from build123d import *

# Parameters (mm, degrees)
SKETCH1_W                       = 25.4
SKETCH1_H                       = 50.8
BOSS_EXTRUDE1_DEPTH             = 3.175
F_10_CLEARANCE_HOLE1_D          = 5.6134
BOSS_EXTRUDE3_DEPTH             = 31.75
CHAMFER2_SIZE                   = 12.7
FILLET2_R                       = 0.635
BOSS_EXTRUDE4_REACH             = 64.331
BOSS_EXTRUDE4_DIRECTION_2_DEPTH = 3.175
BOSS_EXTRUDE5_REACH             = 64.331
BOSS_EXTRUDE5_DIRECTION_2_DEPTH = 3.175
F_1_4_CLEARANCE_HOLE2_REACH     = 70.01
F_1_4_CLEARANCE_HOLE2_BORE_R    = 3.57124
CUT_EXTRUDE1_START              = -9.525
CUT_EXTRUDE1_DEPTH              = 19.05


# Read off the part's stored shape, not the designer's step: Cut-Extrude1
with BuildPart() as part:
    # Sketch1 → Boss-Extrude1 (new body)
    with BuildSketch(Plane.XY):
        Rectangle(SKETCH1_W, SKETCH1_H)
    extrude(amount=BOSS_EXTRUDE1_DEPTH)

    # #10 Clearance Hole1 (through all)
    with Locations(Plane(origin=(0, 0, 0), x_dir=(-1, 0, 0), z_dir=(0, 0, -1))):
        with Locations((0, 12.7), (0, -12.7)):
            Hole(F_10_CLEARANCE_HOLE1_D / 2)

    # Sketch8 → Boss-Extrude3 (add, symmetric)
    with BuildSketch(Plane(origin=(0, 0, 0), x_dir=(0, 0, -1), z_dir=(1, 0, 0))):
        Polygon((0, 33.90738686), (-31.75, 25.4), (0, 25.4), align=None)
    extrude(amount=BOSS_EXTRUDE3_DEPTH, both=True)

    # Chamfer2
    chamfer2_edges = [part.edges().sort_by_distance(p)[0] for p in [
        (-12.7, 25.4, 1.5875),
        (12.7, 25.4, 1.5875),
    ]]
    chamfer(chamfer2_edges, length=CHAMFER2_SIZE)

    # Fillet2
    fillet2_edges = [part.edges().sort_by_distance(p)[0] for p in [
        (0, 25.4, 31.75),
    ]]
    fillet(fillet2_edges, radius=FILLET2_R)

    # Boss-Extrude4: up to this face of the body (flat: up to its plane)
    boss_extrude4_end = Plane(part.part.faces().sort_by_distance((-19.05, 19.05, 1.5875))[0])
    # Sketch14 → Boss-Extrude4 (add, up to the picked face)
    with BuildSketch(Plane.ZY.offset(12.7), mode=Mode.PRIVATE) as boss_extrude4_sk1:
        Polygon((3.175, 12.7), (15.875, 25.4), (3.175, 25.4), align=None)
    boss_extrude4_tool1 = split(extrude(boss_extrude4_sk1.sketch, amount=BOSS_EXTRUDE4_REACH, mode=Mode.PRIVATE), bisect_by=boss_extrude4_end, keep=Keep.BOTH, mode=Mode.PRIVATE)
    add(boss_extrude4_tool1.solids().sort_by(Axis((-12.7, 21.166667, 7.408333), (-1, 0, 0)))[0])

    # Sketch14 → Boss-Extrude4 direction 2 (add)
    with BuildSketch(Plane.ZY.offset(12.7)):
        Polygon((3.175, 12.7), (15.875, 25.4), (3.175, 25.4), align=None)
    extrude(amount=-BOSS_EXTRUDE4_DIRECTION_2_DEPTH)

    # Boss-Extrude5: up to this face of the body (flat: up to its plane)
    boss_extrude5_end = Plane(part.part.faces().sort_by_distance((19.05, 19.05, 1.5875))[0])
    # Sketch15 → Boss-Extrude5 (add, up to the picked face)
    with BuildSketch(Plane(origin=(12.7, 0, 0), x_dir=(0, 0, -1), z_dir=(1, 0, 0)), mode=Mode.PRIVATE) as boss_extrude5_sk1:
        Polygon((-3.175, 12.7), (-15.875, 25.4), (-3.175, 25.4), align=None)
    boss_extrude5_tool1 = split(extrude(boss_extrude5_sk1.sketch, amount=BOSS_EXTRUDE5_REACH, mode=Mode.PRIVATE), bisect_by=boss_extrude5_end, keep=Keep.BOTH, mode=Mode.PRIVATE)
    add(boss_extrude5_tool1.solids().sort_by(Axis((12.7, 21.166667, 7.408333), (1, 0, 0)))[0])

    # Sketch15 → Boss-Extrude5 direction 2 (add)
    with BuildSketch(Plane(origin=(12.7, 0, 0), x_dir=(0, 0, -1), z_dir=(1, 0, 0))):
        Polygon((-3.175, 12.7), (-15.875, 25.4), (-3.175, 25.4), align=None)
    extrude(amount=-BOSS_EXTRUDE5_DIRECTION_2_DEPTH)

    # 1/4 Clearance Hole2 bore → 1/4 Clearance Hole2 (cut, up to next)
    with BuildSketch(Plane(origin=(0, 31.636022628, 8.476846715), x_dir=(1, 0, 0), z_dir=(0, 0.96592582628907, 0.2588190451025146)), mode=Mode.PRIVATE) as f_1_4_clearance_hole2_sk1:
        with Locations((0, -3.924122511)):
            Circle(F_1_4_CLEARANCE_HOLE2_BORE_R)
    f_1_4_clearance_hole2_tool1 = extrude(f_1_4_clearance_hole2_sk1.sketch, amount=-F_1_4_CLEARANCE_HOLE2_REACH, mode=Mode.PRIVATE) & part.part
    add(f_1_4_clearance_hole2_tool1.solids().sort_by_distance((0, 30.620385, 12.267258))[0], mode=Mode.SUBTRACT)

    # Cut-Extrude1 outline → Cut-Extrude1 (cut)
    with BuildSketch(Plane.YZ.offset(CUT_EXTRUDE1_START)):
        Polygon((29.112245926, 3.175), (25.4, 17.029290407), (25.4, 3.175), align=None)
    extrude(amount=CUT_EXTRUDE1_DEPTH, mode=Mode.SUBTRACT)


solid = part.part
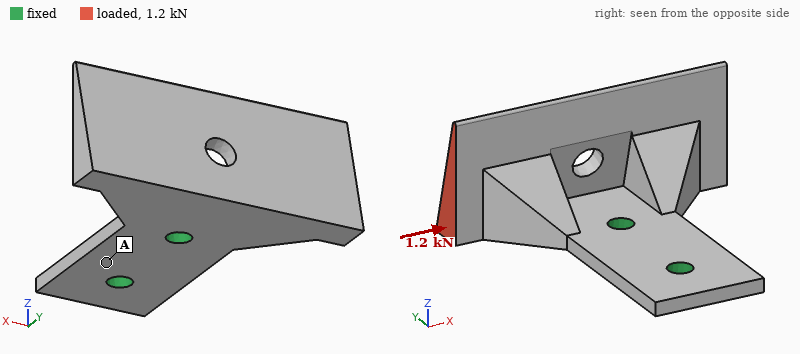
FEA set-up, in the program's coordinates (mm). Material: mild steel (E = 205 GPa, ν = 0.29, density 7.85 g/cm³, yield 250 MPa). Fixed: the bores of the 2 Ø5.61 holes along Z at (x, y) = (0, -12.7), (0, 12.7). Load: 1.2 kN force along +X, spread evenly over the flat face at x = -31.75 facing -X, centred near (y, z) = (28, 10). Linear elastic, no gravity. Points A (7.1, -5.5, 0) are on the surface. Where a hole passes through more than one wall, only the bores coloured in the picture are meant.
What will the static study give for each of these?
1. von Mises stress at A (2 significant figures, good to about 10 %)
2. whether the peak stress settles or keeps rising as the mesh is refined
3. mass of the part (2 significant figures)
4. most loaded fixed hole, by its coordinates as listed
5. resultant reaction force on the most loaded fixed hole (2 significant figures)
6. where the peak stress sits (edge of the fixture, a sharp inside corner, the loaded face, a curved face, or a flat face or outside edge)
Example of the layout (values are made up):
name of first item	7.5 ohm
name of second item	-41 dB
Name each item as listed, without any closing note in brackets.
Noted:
von Mises stress at A	28 MPa
whether the peak stress settles or keeps rising as the mesh is refined	keeps rising
mass of the part	110 g
most loaded fixed hole, by its coordinates as listed	(0, 12.7)
resultant reaction force on the most loaded fixed hole	1.7 kN
where the peak stress sits	edge of the fixture
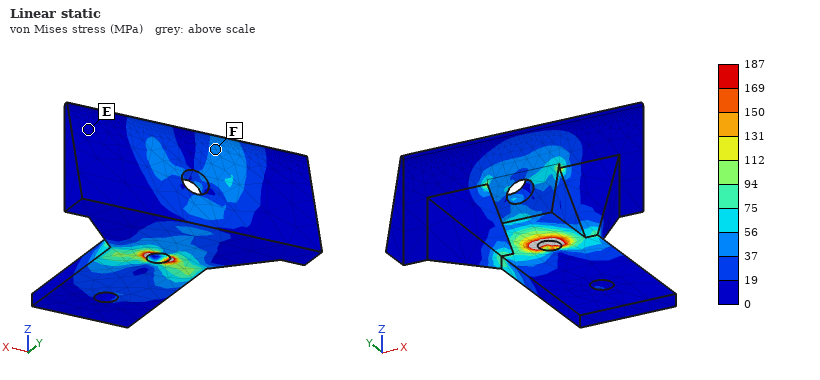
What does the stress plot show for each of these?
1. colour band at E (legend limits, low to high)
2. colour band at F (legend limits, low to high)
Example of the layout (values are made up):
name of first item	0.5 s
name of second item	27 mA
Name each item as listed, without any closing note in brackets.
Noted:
colour band at E	0 to 19 MPa
colour band at F	37 to 56 MPa
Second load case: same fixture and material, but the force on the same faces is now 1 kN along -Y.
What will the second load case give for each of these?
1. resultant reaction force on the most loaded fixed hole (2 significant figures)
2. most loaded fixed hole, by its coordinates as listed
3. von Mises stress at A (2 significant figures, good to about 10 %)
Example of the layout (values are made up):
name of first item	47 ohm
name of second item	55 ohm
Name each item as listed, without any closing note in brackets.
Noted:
resultant reaction force on the most loaded fixed hole	1.1 kN
most loaded fixed hole, by its coordinates as listed	(0, 12.7)
von Mises stress at A	14 MPa
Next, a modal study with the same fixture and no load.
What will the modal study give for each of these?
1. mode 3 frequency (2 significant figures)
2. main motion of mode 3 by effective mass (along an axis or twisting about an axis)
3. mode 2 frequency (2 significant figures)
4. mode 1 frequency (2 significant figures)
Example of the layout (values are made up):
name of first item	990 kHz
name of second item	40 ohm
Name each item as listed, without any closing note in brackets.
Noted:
mode 3 frequency	5100 Hz
main motion of mode 3 by effective mass	along X
mode 2 frequency	2000 Hz
mode 1 frequency	1600 Hz
